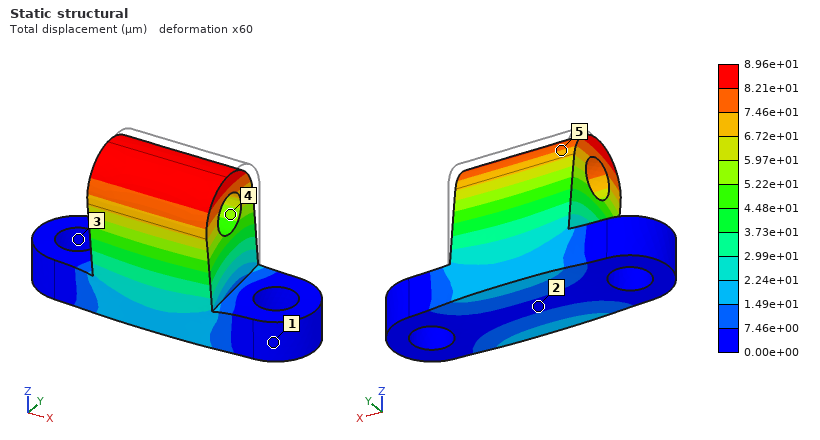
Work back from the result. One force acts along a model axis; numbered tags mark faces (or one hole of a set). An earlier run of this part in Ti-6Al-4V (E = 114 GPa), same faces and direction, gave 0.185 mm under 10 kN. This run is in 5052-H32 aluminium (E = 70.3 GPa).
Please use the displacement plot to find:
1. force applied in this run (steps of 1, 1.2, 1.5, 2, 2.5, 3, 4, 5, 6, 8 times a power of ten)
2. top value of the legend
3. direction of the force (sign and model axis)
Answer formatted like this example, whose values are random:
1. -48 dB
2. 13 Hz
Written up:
1. 3 kN
2. 8.96e+01 µm
3. -Y
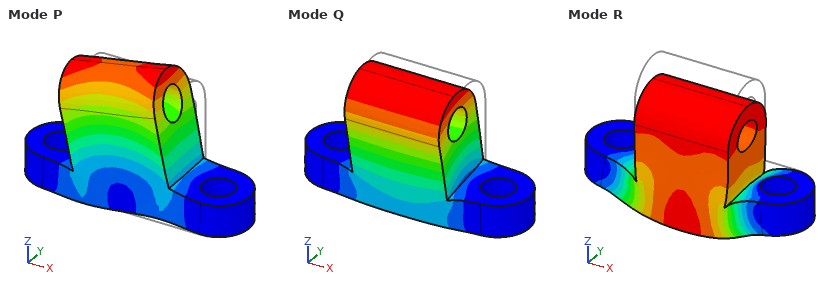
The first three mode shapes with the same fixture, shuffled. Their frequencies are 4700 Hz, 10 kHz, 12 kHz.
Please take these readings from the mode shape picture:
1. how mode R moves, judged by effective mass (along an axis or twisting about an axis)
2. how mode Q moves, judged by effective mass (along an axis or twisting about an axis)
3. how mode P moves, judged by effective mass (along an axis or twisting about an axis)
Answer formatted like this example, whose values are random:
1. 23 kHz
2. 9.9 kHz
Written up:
1. along Z
2. along Y
3. along X
